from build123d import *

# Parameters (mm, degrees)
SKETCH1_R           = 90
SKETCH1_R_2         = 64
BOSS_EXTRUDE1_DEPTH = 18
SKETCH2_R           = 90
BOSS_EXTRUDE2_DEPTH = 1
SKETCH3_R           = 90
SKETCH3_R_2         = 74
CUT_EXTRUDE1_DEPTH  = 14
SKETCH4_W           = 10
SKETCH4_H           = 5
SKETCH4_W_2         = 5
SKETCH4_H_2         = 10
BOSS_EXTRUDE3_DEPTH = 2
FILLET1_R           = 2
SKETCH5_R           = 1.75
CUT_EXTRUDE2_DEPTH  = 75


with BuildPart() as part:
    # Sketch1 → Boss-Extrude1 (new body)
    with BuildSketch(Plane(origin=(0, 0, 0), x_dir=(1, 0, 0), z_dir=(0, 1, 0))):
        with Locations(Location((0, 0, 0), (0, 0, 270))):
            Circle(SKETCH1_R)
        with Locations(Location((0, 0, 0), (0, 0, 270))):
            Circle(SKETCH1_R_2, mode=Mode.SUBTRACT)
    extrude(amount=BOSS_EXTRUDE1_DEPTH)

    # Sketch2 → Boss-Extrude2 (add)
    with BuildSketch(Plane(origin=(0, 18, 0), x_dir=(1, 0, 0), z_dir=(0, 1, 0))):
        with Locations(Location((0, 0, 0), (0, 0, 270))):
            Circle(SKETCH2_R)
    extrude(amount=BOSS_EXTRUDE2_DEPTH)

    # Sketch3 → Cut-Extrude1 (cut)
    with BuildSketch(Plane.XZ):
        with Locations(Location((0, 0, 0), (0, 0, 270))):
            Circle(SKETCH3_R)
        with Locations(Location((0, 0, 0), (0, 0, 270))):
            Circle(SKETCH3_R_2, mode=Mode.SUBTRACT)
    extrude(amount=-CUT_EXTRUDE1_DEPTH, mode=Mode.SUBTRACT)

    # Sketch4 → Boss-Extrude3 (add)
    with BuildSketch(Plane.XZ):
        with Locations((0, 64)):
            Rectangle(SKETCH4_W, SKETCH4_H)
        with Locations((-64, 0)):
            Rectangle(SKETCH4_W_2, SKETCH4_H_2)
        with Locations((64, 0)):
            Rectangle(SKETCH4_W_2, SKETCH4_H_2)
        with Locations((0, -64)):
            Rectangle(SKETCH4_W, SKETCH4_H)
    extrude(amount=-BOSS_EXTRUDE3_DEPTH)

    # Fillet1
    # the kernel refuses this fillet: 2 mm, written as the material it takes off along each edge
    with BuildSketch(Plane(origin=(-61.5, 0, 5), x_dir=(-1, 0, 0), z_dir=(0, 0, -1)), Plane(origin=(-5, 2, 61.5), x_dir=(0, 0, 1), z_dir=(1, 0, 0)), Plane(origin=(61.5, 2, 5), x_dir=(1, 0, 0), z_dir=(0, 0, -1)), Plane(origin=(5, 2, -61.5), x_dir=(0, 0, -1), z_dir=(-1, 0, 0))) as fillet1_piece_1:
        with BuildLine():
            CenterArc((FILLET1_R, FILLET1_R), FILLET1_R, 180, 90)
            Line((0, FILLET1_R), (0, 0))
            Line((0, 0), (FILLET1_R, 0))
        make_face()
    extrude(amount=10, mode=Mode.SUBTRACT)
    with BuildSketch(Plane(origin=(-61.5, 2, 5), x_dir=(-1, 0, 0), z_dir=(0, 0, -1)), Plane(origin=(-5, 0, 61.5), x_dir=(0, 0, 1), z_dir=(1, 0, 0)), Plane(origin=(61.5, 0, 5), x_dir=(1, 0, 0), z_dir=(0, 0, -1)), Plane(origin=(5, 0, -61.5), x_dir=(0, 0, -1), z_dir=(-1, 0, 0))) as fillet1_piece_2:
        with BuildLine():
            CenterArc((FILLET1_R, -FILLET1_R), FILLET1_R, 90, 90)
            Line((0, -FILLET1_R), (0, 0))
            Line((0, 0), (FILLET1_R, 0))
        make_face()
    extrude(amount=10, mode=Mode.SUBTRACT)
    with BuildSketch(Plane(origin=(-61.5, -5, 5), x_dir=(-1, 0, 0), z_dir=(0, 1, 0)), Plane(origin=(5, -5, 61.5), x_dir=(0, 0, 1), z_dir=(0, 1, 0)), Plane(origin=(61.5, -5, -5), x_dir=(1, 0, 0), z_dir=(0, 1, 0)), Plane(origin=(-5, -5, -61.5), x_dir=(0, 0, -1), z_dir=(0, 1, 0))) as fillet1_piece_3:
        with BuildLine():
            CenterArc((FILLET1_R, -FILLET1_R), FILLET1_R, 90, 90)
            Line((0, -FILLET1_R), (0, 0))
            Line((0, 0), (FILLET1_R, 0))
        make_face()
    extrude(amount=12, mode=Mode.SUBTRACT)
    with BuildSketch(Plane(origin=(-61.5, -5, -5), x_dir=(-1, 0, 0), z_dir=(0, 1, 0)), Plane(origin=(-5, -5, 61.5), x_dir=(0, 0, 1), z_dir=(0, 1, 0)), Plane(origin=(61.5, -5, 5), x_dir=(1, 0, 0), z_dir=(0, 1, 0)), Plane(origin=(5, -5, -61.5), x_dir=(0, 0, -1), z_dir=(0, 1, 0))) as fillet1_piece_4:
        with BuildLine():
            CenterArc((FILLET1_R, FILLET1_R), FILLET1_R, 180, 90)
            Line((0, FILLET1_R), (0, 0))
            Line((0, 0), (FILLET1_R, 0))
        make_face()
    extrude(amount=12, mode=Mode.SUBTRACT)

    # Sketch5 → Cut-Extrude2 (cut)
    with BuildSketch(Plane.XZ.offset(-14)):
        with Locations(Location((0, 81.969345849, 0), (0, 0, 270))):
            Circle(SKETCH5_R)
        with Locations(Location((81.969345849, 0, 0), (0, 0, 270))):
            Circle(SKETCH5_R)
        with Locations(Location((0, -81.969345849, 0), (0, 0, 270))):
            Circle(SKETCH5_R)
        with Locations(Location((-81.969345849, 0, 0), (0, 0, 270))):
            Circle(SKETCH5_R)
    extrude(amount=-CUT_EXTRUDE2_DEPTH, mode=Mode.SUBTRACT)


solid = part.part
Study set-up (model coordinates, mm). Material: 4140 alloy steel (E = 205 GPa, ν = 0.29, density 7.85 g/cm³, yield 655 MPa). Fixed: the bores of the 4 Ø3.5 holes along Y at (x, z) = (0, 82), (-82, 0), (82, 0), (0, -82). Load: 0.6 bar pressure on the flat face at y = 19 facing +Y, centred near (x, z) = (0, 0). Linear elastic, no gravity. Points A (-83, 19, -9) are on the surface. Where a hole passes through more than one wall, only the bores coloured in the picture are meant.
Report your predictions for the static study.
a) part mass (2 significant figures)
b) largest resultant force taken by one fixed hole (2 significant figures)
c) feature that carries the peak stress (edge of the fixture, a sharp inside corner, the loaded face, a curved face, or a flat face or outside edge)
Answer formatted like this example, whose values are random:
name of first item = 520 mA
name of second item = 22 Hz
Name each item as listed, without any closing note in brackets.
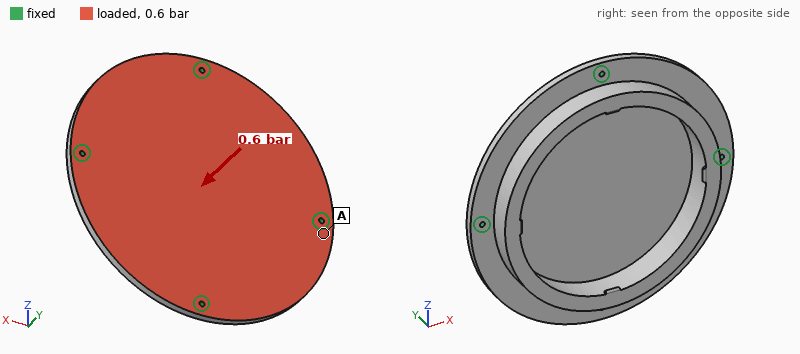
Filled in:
part mass = 1.1 kg
largest resultant force taken by one fixed hole = 420 N
feature that carries the peak stress = the loaded face
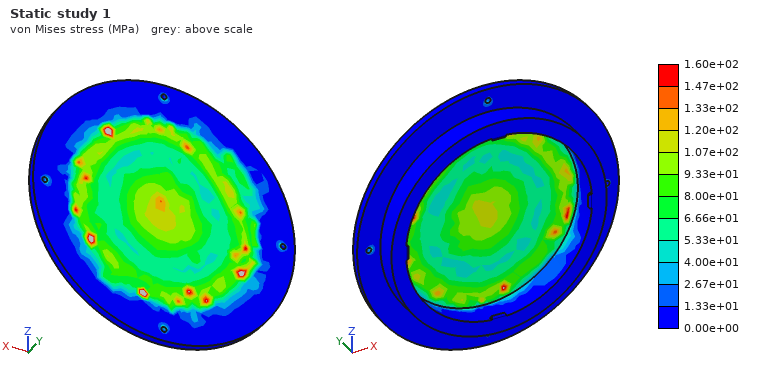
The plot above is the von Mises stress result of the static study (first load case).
